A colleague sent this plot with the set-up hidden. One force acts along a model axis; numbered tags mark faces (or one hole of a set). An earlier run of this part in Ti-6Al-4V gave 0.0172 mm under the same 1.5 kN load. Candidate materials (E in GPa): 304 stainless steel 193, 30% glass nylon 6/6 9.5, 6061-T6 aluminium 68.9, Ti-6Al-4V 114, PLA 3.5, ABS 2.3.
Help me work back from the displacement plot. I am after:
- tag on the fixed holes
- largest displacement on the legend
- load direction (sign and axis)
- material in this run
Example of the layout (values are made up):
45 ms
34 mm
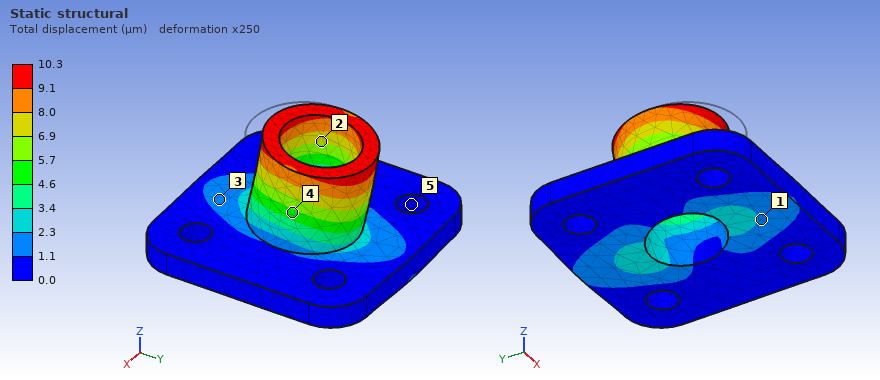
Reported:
5
10.3 µm
+Y
304 stainless steel
